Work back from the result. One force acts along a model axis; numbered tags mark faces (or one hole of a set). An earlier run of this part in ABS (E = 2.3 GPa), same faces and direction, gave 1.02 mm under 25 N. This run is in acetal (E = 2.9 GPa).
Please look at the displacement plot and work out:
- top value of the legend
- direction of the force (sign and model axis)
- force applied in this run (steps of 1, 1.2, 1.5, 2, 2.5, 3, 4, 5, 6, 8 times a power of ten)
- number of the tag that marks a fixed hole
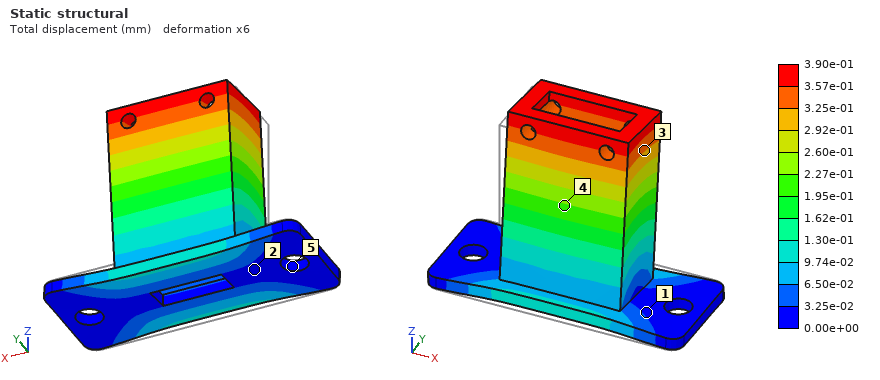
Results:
3.90e-01 mm
+Y
12 N
5
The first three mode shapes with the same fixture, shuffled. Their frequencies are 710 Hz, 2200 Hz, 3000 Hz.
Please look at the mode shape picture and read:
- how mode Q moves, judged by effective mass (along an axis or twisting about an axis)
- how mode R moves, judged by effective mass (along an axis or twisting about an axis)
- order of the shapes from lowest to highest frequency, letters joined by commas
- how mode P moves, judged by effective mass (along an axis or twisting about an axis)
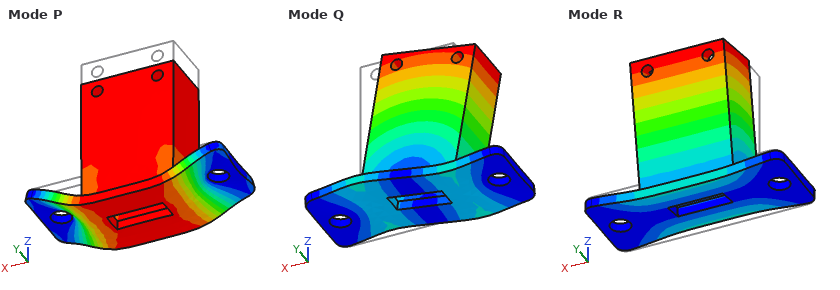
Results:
along X
along Y
R, Q, P
along Z
